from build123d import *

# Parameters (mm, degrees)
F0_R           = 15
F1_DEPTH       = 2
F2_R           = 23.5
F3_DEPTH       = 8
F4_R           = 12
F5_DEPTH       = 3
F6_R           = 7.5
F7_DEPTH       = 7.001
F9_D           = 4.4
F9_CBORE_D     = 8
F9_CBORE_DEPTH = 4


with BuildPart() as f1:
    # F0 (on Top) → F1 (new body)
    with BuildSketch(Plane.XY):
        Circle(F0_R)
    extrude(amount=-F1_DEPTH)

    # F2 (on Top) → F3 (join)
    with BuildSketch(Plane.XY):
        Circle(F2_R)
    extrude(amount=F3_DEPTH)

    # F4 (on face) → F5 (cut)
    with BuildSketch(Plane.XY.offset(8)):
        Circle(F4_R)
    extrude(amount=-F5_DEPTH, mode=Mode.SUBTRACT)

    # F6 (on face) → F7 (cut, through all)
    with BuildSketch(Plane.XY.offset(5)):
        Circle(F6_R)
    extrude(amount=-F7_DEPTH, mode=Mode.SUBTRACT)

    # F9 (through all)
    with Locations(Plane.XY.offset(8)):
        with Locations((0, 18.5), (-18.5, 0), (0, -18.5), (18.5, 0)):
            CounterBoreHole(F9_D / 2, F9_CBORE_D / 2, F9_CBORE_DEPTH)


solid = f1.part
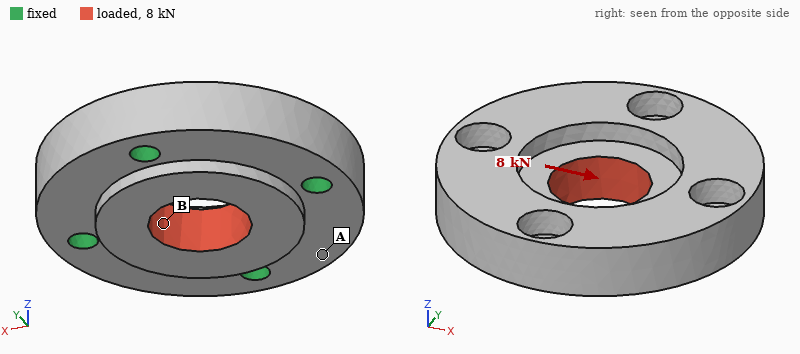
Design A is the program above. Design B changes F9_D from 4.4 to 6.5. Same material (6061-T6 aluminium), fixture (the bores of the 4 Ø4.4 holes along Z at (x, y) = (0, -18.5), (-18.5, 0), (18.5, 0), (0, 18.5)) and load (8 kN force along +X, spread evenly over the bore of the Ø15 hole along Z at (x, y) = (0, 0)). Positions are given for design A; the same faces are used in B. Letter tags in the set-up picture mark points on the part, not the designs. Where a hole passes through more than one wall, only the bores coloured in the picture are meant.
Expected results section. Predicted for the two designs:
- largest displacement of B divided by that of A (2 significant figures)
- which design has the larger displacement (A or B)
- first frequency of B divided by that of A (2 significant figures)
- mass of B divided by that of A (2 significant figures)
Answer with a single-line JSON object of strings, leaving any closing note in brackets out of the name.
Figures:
{"largest displacement of B divided by that of A": "0.85", "which design has the larger displacement": "A", "first frequency of B divided by that of A": "1.3", "mass of B divided by that of A": "0.98"}
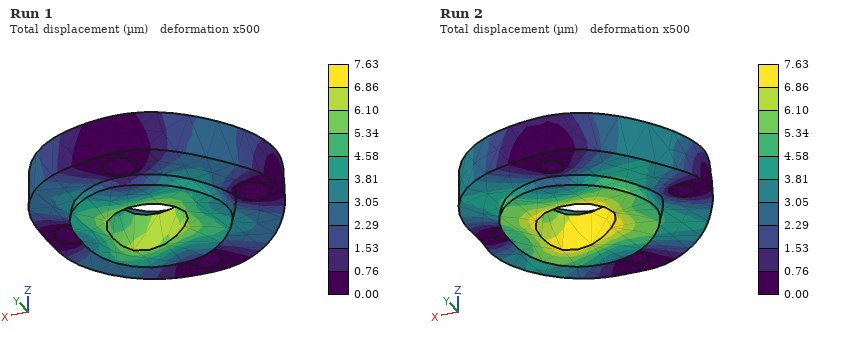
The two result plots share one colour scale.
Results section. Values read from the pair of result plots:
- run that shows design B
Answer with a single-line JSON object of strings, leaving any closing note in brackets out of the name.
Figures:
{"run that shows design B": "Run 1"}
